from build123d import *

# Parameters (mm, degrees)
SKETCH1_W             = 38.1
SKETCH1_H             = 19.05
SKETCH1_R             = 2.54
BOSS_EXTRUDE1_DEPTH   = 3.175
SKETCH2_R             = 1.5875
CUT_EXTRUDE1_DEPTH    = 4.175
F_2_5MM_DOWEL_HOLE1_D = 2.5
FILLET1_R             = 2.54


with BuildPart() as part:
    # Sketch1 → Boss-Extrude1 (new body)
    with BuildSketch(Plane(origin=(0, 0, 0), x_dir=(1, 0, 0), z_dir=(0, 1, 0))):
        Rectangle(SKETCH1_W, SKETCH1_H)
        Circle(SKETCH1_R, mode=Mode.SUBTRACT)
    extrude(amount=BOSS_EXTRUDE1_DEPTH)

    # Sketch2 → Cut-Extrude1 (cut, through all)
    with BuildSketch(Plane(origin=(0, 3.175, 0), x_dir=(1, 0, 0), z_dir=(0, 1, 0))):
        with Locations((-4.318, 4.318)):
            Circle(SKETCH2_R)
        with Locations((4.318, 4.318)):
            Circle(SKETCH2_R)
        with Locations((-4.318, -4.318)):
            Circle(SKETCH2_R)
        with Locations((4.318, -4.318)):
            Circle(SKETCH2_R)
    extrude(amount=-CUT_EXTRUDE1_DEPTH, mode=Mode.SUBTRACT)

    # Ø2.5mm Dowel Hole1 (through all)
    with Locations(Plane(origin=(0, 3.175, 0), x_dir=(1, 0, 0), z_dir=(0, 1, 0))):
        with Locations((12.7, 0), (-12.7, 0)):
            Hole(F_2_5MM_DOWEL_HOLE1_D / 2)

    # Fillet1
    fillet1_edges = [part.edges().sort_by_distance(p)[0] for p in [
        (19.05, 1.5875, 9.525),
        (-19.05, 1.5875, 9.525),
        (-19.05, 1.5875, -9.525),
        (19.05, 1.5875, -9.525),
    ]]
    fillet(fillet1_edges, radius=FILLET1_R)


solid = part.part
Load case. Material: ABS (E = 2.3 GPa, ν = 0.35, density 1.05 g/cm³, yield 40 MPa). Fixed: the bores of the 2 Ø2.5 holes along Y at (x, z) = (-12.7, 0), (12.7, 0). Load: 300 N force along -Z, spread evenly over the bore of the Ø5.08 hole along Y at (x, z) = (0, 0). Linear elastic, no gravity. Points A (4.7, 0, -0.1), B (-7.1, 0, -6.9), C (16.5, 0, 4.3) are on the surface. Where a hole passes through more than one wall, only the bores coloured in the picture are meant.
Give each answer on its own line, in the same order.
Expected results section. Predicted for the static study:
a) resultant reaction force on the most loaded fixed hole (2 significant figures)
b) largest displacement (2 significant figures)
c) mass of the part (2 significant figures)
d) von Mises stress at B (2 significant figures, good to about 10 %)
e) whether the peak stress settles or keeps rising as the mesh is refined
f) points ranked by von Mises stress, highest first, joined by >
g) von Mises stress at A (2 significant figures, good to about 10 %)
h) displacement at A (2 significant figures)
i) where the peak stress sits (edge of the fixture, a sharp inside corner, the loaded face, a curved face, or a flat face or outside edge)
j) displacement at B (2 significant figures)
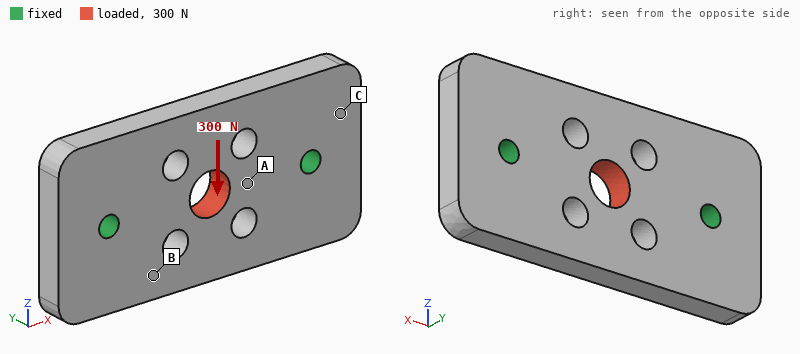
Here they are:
150 N
79 µm
2.2 g
4.9 MPa
keeps rising
A > B > C
9.3 MPa
56 µm
edge of the fixture
37 µm
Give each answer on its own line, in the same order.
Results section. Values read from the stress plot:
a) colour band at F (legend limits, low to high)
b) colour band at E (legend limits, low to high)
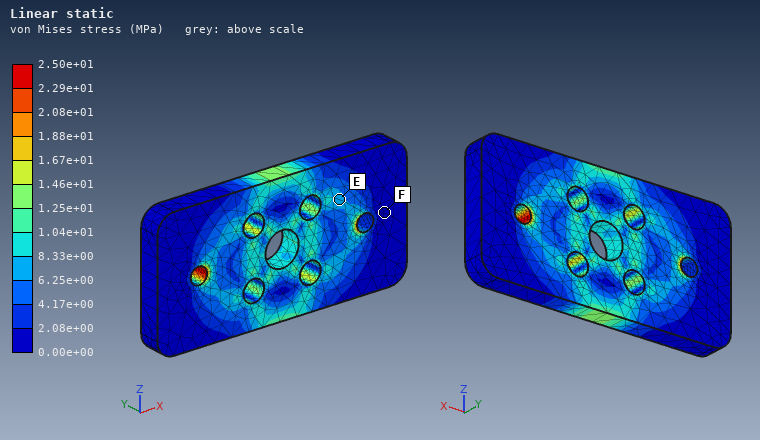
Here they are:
0.00e+00 to 2.08e+00 MPa
6.25e+00 to 8.33e+00 MPa
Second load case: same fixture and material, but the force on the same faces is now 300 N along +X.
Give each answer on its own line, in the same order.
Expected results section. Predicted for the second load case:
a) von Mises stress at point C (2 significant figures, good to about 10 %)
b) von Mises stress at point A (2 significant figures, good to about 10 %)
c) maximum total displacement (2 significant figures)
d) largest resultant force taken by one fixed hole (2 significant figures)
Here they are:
1.3 MPa
5.3 MPa
35 µm
150 N
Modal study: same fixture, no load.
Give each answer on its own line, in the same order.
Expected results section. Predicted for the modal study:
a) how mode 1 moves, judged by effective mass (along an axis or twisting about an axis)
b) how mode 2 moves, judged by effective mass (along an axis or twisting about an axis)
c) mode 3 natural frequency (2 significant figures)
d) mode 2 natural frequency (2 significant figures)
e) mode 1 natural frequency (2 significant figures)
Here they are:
twisting about X
along Y
7500 Hz
5400 Hz
4900 Hz
